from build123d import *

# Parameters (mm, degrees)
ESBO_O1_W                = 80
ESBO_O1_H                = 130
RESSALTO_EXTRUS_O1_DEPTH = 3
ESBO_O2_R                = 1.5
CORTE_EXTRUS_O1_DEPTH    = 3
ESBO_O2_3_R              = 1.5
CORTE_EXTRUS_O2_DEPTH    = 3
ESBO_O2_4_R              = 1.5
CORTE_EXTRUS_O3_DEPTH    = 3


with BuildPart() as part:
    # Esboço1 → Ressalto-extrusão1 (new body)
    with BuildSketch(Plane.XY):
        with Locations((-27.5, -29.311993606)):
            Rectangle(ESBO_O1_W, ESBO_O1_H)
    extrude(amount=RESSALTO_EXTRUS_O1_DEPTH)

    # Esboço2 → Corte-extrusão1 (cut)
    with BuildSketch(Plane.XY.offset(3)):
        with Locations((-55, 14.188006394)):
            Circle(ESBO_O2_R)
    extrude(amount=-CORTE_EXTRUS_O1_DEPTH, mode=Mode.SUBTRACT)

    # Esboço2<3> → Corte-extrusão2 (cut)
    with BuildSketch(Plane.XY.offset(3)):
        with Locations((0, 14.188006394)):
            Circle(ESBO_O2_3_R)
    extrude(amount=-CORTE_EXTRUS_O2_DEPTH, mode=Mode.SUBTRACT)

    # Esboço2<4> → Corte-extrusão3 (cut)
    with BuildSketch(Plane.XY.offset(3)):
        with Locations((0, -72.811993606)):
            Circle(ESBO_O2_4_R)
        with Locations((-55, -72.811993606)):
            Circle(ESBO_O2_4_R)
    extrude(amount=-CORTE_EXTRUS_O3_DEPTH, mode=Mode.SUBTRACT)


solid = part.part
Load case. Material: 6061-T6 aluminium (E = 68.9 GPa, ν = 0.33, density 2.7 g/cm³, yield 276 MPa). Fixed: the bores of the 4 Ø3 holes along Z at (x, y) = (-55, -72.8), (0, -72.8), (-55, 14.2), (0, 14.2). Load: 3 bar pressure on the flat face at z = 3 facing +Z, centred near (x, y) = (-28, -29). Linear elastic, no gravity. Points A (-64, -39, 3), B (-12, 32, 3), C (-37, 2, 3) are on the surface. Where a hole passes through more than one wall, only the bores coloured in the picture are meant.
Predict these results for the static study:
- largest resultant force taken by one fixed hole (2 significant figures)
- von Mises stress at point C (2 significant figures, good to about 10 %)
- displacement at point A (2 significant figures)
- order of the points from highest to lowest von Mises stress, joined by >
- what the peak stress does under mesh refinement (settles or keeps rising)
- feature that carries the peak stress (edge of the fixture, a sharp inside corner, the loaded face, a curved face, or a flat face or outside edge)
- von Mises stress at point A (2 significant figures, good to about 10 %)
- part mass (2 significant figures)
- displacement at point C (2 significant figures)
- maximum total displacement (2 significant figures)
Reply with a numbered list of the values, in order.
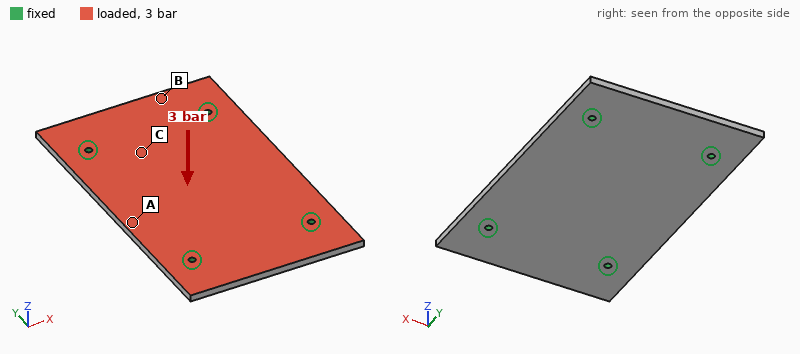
1. 780 N
2. 35 MPa
3. 0.32 mm
4. A > C > B
5. keeps rising
6. edge of the fixture
7. 64 MPa
8. 84 g
9. 0.17 mm
10. 0.39 mm
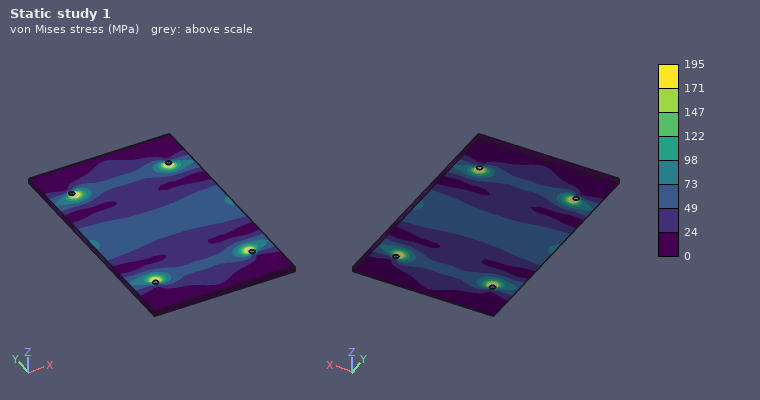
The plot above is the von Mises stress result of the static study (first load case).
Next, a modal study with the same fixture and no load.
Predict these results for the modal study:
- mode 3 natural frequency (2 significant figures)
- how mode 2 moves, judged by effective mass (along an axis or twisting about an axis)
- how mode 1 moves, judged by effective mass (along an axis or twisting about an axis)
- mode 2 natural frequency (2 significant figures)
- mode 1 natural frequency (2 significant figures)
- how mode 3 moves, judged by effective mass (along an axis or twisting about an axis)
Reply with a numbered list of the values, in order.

1. 3300 Hz
2. twisting about Y
3. along Z
4. 2400 Hz
5. 1700 Hz
6. along Z
